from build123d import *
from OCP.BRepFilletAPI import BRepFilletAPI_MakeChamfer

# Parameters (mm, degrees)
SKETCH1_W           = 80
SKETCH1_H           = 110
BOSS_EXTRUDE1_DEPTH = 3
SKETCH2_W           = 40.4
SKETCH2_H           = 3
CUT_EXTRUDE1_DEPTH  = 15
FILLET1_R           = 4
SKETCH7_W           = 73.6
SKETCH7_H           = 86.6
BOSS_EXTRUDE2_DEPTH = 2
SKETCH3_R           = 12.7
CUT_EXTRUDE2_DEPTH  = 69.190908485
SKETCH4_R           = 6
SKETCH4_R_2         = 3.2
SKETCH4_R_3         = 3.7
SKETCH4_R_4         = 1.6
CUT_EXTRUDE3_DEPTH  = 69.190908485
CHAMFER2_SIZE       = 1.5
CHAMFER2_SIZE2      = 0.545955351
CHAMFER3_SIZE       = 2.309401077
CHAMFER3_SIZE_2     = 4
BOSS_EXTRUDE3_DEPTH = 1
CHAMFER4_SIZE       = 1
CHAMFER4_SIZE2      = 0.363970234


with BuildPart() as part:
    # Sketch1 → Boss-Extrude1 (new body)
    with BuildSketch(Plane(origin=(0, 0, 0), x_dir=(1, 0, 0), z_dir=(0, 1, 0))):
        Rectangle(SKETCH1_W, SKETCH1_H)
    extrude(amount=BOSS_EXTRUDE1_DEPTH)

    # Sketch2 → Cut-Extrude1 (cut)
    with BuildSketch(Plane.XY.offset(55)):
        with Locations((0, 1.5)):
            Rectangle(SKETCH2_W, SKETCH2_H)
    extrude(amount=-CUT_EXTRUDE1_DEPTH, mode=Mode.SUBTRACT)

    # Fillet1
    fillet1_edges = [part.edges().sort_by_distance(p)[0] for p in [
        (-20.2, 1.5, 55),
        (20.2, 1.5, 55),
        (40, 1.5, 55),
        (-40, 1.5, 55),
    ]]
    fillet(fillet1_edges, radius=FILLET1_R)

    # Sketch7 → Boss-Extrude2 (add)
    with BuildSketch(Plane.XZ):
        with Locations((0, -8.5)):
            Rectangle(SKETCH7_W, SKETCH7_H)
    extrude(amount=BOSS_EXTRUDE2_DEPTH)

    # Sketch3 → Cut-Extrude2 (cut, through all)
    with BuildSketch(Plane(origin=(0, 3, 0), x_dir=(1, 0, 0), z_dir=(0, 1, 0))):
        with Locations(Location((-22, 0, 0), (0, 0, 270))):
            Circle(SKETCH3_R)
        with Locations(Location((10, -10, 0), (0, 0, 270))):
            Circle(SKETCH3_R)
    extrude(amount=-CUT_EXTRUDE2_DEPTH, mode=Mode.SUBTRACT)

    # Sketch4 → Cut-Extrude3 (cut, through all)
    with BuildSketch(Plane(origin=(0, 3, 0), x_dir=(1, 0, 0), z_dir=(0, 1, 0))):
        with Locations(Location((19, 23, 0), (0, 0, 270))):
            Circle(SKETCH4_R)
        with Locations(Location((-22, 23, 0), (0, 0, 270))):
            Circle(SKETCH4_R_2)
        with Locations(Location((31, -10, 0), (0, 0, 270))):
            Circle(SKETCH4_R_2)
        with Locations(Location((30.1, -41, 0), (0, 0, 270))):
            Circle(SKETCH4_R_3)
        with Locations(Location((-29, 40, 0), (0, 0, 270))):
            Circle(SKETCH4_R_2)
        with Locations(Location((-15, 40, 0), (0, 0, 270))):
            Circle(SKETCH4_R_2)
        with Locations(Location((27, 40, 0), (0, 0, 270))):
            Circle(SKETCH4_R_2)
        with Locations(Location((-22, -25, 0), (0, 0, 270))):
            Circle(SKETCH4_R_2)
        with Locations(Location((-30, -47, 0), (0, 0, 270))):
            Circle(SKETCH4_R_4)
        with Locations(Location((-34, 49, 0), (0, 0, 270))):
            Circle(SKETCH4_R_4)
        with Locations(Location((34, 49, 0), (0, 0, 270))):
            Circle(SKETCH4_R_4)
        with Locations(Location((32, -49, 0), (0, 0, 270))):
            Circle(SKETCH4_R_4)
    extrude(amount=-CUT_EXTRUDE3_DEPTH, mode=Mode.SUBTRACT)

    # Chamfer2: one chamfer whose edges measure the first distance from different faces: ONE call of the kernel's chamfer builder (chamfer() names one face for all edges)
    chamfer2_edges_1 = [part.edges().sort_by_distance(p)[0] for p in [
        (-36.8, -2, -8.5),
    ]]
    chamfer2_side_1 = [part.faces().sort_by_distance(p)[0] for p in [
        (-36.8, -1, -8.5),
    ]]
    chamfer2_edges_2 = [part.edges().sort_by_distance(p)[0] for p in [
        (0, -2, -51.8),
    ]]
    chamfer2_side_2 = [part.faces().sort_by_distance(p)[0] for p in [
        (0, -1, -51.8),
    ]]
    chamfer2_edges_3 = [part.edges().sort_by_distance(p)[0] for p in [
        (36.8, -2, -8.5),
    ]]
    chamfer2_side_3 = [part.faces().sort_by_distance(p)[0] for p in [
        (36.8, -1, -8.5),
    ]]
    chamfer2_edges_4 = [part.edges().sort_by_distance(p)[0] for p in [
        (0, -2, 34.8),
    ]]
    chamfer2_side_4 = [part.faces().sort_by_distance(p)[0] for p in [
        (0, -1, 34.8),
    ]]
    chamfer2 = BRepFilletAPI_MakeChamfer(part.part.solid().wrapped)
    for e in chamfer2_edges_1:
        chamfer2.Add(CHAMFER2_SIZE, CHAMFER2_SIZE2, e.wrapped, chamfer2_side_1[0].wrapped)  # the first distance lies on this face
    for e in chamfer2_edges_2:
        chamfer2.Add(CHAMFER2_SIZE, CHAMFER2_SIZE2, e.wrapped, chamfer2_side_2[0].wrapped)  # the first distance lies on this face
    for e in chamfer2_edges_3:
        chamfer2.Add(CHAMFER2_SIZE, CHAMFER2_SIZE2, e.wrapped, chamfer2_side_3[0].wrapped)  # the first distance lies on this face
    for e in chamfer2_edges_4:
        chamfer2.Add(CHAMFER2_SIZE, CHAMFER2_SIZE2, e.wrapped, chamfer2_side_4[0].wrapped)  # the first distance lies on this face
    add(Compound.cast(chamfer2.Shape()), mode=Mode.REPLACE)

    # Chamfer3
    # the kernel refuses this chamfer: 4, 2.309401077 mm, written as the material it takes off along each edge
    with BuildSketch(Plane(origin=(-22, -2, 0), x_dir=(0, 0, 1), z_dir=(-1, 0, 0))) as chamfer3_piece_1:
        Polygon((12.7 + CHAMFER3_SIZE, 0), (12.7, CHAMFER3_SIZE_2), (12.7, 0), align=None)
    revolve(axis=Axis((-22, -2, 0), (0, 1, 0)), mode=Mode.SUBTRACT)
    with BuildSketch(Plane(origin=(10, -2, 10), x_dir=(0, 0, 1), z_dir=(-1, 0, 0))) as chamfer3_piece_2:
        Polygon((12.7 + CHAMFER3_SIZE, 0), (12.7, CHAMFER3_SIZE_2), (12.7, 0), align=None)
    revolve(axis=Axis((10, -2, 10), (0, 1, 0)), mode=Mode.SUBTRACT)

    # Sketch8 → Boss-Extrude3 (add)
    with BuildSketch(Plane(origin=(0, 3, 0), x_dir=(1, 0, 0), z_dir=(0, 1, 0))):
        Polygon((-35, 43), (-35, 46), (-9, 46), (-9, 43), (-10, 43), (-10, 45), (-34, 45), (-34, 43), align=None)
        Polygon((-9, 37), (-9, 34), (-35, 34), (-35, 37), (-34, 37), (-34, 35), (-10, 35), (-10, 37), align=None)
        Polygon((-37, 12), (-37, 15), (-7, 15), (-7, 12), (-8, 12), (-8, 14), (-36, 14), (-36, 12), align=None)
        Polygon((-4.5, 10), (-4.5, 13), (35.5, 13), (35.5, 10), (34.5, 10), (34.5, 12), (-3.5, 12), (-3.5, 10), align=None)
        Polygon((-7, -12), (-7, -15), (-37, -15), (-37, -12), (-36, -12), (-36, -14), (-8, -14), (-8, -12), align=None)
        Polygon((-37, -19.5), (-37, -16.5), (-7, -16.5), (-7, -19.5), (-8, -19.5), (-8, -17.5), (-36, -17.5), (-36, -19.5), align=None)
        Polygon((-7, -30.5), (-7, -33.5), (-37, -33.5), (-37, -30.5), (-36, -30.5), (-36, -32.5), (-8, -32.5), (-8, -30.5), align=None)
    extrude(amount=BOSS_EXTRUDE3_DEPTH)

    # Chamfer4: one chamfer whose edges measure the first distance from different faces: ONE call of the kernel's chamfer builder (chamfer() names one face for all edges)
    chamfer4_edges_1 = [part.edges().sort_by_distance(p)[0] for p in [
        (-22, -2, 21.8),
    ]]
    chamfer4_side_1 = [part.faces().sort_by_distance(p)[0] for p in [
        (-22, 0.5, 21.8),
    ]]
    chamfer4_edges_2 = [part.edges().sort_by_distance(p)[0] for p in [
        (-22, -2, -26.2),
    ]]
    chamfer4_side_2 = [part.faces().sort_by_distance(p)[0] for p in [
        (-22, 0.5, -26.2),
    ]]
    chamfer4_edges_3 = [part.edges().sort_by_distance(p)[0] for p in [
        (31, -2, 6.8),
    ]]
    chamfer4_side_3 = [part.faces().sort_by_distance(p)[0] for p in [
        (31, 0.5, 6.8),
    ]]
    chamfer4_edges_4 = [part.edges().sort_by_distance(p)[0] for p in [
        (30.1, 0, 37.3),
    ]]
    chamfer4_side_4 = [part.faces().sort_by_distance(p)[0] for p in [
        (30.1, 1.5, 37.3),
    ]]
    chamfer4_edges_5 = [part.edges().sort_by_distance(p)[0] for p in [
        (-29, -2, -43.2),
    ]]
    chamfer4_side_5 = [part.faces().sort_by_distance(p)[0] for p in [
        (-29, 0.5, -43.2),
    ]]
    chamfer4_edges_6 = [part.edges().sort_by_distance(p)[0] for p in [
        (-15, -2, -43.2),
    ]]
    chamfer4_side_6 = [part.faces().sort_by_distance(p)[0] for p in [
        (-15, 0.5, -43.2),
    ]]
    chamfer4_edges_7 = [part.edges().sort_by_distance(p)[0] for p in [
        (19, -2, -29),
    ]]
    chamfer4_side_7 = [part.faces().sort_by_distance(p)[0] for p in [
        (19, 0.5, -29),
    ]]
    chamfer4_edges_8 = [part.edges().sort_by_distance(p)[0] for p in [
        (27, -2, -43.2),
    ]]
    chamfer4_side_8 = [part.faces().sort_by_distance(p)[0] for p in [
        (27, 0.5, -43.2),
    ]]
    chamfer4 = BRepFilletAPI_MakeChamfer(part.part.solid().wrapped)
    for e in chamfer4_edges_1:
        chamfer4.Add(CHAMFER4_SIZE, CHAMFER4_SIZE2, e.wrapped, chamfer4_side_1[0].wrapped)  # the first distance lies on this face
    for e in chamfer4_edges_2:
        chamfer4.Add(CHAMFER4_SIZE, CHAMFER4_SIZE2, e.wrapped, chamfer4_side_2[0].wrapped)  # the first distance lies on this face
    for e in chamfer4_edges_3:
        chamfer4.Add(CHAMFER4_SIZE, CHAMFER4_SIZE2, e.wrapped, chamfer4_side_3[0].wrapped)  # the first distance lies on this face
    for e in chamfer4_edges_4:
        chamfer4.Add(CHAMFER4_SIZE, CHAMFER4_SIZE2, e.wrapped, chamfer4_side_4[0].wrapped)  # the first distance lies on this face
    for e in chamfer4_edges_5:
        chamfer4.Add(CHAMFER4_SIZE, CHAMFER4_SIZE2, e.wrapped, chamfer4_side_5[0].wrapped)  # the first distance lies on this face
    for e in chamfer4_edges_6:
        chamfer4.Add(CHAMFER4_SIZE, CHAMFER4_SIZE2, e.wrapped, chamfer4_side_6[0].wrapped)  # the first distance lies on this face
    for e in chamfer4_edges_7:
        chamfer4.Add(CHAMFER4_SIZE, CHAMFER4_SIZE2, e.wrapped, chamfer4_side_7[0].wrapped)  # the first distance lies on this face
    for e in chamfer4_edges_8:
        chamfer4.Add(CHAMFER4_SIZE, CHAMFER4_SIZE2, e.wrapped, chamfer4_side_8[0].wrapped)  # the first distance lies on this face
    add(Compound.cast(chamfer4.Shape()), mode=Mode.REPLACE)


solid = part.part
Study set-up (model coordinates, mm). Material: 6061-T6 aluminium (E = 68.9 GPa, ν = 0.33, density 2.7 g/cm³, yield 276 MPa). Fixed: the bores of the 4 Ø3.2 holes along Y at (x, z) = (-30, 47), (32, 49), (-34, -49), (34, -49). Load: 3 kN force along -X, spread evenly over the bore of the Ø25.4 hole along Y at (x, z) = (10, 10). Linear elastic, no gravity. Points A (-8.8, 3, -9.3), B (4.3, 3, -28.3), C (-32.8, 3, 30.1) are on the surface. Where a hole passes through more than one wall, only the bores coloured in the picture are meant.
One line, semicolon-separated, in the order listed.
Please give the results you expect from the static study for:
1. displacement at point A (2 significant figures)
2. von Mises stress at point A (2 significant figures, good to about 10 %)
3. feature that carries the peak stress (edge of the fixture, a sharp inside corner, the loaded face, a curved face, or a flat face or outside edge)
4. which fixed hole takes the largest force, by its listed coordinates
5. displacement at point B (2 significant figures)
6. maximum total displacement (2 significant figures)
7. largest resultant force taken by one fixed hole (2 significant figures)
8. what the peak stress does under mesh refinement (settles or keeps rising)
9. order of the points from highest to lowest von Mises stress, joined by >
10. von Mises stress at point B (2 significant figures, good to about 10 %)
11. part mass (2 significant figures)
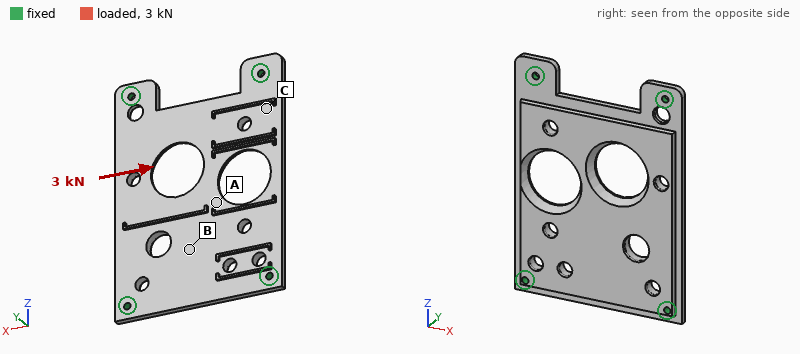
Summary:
27 µm; 23 MPa; edge of the fixture; (-34, -49); 10 µm; 52 µm; 1.2 kN; keeps rising; A > B > C; 14 MPa; 80 g
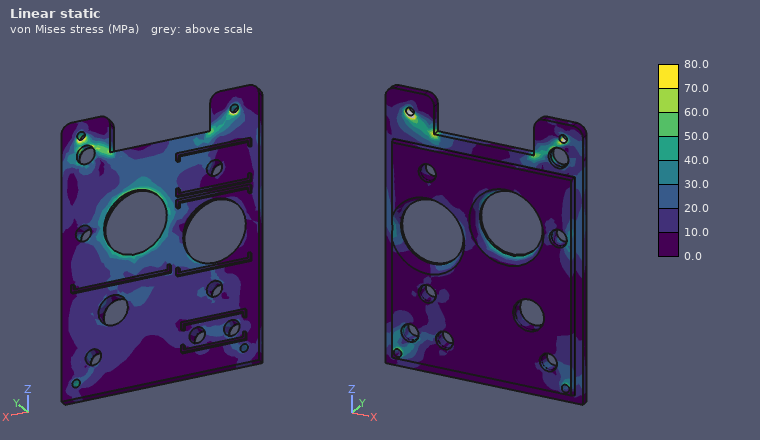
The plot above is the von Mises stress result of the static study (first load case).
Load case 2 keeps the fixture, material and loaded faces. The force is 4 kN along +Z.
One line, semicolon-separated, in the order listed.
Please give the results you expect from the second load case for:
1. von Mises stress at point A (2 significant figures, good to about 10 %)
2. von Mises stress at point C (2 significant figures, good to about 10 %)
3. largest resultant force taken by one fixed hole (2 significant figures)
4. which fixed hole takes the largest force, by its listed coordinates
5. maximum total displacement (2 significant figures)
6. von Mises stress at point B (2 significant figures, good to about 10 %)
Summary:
25 MPa; 8.9 MPa; 1.4 kN; (34, -49); 40 µm; 8.6 MPa
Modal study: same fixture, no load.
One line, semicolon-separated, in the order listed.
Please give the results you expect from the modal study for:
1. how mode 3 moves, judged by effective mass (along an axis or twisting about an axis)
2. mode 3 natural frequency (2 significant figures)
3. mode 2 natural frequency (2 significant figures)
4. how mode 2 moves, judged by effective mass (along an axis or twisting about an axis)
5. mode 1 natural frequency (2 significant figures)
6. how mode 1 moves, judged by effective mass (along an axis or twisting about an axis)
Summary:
twisting about X; 4000 Hz; 2800 Hz; twisting about Z; 1600 Hz; along Y
